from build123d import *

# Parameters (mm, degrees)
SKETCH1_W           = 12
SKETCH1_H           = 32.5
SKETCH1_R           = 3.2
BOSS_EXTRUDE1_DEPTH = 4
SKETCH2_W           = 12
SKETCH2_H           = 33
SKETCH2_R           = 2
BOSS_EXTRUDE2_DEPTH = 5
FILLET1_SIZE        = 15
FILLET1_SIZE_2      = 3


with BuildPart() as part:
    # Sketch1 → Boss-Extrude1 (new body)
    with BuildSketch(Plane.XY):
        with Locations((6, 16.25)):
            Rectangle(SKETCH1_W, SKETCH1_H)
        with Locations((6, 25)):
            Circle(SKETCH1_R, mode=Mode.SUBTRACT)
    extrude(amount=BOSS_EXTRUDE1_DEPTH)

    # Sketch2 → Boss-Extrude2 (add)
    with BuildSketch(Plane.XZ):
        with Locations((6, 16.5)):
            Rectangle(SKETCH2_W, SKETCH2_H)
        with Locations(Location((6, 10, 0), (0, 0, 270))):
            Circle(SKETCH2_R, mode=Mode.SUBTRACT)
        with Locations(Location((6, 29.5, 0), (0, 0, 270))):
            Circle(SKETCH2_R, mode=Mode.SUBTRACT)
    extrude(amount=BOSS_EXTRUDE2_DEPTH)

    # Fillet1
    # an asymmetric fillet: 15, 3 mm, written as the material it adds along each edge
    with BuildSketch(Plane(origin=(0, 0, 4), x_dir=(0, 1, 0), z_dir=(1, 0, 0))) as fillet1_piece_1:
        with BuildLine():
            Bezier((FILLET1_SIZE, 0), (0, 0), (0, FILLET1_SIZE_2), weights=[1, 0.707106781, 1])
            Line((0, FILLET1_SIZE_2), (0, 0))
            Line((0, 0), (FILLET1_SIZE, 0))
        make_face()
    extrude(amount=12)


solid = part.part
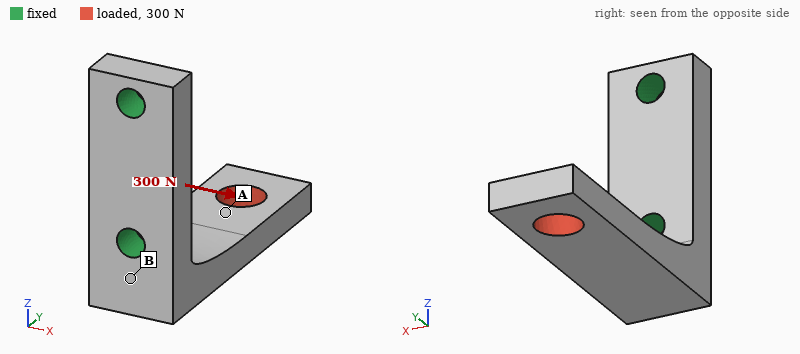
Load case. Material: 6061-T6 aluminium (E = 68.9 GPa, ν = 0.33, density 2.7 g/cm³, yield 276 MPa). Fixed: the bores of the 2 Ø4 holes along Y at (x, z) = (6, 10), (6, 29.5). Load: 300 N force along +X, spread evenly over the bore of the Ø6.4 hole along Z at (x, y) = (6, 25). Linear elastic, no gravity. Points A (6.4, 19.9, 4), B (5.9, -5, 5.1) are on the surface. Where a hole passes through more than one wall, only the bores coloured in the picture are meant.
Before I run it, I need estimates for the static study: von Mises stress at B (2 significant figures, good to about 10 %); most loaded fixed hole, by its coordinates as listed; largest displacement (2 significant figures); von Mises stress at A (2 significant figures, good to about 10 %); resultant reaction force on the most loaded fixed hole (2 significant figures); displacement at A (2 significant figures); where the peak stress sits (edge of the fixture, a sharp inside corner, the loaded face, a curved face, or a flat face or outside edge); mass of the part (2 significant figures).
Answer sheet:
72 MPa
(6, 10)
0.19 mm
28 MPa
350 N
0.11 mm
edge of the fixture
9.2 g
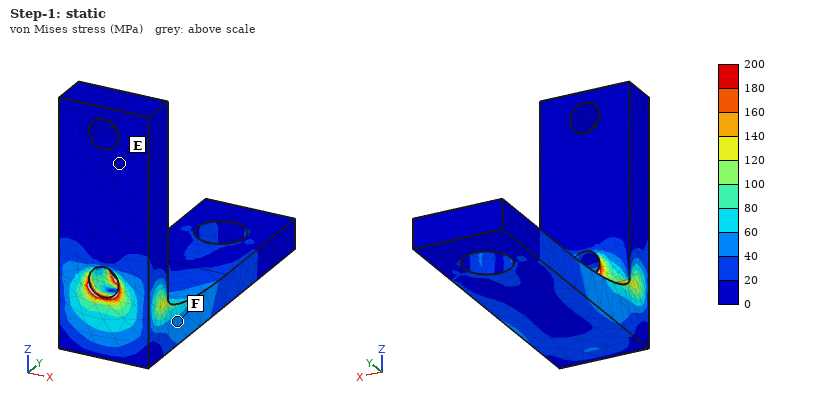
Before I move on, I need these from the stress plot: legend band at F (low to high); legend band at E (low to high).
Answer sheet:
40 to 60 MPa
0 to 20 MPa
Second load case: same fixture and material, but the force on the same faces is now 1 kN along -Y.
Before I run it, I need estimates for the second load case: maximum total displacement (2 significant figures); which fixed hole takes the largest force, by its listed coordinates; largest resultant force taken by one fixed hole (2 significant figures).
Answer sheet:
0.13 mm
(6, 10)
1.0 kN
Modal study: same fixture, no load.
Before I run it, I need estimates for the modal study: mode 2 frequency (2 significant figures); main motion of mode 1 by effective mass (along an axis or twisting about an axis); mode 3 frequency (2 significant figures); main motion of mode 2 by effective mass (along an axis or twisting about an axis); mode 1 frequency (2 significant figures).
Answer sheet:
5100 Hz
along Z
13 kHz
along X
3200 Hz
